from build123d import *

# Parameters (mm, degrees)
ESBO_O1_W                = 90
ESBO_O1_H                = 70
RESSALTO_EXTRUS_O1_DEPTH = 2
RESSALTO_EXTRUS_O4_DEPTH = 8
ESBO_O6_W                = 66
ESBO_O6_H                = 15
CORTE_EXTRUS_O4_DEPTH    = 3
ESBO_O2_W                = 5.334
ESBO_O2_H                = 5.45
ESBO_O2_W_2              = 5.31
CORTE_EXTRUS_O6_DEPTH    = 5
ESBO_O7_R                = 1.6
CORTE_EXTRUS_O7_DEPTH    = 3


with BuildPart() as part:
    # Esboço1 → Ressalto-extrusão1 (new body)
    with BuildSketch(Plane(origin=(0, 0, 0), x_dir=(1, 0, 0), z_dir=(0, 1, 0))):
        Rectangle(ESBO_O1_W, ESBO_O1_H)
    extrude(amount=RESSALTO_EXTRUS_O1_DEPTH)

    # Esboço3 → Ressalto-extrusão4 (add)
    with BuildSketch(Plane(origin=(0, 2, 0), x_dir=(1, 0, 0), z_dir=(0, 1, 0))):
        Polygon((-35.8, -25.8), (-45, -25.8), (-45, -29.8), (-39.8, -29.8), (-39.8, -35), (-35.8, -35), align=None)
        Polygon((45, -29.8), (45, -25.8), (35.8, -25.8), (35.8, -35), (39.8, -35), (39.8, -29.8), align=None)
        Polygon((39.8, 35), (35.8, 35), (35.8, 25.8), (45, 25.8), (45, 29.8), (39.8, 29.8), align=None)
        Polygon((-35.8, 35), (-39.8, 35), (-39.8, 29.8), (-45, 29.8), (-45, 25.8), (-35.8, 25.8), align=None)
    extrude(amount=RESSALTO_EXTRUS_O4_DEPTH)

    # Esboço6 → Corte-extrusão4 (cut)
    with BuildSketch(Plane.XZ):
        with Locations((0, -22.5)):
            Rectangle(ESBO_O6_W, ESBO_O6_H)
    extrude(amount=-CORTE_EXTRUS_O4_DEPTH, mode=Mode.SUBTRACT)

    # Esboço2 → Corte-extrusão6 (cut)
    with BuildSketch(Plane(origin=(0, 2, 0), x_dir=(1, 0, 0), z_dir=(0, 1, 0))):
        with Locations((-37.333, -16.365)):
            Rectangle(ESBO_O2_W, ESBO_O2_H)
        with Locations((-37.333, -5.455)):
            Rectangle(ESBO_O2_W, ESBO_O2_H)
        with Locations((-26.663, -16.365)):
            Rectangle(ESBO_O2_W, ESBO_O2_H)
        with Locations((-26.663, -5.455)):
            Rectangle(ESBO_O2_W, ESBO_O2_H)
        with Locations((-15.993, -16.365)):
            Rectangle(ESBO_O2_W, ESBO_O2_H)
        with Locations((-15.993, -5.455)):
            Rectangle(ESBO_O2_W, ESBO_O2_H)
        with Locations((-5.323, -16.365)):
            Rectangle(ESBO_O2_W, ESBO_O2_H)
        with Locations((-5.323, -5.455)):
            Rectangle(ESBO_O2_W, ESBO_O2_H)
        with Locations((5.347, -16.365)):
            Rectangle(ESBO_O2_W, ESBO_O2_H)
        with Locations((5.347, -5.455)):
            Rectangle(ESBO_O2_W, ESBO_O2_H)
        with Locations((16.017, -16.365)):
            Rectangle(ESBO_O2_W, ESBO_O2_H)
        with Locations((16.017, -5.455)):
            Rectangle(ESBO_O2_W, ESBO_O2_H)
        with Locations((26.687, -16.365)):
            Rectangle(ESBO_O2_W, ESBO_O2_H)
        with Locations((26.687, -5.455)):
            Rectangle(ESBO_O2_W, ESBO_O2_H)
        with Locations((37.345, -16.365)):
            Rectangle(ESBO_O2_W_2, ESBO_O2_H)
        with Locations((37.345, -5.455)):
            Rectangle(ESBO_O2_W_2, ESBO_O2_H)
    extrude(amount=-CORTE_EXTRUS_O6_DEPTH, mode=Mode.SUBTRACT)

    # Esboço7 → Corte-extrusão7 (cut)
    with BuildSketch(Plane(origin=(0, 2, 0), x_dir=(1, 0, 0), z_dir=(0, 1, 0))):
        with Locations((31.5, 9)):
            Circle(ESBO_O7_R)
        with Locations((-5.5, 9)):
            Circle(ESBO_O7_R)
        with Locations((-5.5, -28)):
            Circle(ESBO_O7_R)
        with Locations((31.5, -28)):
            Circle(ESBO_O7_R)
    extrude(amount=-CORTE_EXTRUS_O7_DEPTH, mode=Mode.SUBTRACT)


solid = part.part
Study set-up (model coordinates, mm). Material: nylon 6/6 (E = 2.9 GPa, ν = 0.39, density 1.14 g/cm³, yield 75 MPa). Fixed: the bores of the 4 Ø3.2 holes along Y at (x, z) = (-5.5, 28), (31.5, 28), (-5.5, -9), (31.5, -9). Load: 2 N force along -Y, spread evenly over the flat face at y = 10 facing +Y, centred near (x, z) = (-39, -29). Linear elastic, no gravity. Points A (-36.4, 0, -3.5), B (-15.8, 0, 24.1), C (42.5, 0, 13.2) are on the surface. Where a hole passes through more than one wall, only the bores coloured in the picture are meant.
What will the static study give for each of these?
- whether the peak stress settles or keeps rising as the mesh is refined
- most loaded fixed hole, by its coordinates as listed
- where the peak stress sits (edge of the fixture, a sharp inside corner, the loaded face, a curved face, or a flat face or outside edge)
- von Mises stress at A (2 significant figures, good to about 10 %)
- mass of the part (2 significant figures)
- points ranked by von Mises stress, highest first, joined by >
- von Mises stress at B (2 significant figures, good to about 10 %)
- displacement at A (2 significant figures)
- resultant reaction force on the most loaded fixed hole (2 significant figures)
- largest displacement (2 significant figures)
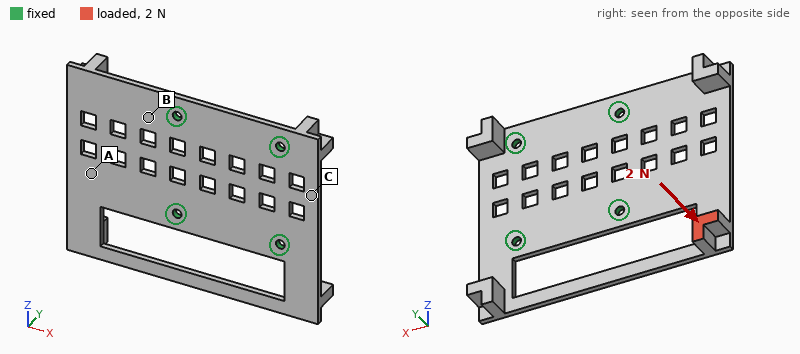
keeps rising
(-5.5, -9)
edge of the fixture
2.1 MPa
13 g
A > B > C
0.90 MPa
0.35 mm
3.0 N
1.3 mm
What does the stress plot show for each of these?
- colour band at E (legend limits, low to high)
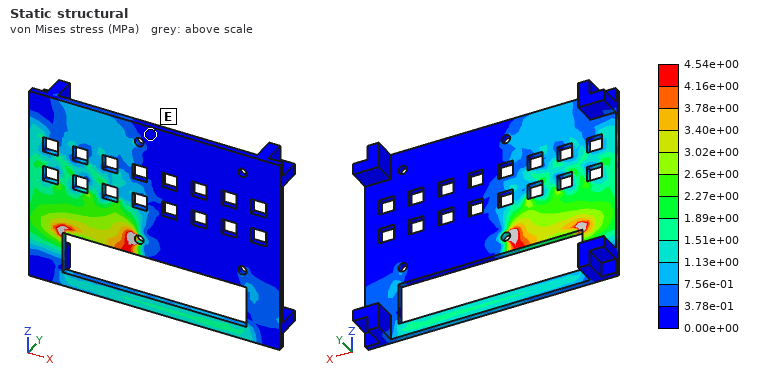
0.00e+00 to 3.78e-01 MPa
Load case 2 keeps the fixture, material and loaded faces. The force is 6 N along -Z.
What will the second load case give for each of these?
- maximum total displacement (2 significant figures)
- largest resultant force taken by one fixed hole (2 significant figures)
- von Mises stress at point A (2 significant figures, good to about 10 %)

1.1 mm
5.4 N
2.0 MPa
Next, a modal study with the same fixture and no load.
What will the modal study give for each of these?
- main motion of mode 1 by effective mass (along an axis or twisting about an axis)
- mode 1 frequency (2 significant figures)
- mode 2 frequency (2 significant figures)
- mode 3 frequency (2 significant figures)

along Y
190 Hz
290 Hz
390 Hz
